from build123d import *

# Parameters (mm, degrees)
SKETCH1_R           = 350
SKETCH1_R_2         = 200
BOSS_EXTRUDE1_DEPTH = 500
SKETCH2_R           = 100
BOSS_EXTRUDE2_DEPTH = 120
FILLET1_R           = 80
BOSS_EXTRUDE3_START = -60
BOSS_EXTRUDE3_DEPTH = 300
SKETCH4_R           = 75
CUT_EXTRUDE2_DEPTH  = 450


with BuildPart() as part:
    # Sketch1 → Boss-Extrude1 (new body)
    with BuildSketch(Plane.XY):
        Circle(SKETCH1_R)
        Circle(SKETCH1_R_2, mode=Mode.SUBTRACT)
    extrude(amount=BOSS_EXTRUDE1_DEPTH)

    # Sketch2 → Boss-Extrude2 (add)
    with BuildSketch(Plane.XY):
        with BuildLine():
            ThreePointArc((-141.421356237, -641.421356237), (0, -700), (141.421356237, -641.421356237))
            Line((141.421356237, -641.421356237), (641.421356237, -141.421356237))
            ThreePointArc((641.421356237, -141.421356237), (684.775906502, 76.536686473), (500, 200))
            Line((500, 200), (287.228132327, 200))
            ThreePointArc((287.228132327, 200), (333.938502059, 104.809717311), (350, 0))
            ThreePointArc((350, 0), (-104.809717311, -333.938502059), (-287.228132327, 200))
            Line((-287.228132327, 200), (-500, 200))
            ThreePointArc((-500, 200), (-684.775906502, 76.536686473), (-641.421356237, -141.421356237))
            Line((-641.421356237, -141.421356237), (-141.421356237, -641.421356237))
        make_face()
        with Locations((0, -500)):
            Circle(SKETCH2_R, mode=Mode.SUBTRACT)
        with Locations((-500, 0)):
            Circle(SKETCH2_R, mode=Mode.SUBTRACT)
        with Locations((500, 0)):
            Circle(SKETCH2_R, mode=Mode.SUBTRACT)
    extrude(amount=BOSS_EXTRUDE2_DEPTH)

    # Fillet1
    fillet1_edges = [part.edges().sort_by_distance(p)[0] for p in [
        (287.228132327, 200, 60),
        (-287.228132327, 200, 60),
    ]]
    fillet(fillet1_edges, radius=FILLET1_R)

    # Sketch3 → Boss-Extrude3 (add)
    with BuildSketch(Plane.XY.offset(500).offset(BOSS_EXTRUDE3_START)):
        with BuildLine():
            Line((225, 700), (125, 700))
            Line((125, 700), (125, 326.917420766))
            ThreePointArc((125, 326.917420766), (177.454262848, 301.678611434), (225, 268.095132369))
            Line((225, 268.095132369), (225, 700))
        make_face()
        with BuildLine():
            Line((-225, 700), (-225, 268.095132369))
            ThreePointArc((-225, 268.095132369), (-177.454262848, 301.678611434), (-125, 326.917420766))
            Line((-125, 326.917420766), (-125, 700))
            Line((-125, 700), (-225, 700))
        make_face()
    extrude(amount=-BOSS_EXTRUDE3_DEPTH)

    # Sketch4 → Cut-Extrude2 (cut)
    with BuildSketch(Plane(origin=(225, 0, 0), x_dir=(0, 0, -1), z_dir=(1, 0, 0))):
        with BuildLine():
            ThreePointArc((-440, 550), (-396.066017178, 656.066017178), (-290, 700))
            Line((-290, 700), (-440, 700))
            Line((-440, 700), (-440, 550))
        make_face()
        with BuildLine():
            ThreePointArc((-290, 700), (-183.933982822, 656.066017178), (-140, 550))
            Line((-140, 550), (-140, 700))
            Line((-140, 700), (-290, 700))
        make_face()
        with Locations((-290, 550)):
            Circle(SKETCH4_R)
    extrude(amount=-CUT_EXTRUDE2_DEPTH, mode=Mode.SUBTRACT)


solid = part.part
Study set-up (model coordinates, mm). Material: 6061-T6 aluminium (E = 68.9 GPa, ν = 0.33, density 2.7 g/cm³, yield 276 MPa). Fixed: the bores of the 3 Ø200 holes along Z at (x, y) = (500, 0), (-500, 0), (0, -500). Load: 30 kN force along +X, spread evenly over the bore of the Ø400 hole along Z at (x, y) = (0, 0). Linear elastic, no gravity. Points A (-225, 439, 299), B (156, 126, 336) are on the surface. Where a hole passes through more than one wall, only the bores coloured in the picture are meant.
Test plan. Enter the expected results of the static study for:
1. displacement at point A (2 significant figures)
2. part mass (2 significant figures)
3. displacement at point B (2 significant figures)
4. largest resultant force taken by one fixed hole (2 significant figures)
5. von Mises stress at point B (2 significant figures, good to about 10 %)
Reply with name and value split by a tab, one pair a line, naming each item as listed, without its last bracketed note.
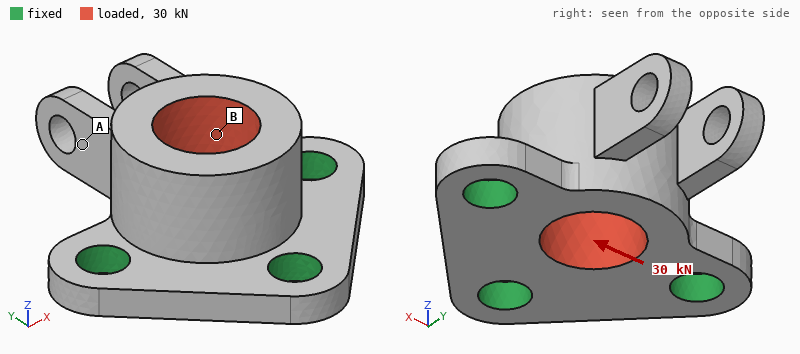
displacement at point A	2.6 µm
part mass	540 kg
displacement at point B	2.7 µm
largest resultant force taken by one fixed hole	14 kN
von Mises stress at point B	0.17 MPa
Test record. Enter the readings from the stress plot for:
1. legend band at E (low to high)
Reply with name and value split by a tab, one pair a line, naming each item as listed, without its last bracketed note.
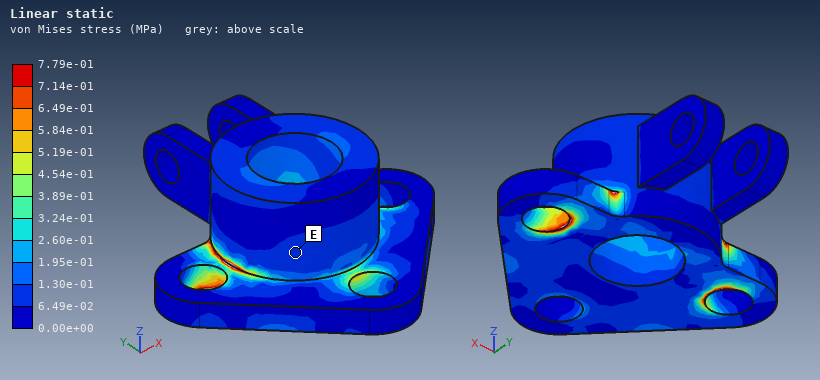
legend band at E	6.49e-02 to 1.30e-01 MPa
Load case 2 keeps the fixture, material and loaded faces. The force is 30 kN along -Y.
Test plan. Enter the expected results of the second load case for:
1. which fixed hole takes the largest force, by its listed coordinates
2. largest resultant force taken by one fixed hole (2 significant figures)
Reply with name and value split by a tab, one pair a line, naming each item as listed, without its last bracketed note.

which fixed hole takes the largest force, by its listed coordinates	(0, -500)
largest resultant force taken by one fixed hole	18 kN
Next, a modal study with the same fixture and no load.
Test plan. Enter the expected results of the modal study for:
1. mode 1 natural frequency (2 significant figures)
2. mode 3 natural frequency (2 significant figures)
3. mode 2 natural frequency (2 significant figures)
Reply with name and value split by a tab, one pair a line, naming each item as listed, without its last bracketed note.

mode 1 natural frequency	360 Hz
mode 3 natural frequency	540 Hz
mode 2 natural frequency	520 Hz
